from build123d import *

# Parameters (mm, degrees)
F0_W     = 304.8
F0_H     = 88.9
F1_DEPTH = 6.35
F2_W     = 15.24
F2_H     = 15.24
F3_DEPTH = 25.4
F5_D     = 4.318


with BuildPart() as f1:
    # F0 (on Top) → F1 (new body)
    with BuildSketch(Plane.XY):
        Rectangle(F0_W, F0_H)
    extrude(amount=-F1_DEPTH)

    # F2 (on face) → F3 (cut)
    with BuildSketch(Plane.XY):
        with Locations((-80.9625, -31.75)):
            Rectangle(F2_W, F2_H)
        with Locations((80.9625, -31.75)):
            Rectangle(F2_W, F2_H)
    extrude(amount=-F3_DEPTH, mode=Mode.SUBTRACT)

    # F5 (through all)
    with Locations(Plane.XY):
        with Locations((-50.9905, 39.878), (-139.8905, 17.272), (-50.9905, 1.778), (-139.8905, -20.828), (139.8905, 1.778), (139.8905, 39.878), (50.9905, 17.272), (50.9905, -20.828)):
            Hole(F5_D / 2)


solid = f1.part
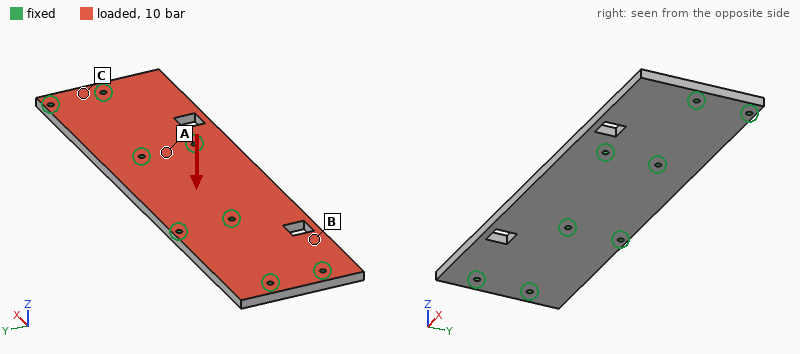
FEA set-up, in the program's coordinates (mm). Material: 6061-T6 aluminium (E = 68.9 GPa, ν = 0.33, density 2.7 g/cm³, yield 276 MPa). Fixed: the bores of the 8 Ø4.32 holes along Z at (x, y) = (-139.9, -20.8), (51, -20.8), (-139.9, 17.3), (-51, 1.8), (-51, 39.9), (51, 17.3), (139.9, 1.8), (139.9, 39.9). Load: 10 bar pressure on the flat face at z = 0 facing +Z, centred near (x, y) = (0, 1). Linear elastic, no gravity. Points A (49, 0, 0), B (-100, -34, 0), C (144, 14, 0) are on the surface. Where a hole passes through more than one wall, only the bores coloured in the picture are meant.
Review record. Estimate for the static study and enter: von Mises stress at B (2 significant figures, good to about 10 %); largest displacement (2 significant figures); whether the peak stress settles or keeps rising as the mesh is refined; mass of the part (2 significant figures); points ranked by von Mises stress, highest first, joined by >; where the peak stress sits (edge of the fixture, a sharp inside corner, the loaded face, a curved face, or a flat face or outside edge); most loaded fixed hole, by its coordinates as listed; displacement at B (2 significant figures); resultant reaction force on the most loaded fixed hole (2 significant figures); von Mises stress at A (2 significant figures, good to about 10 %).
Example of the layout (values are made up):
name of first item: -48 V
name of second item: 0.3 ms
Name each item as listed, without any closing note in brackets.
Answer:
von Mises stress at B: 41 MPa
largest displacement: 0.51 mm
whether the peak stress settles or keeps rising as the mesh is refined: keeps rising
mass of the part: 450 g
points ranked by von Mises stress, highest first, joined by >: A > B > C
where the peak stress sits: edge of the fixture
most loaded fixed hole, by its coordinates as listed: (-51, 1.8)
displacement at B: 0.27 mm
resultant reaction force on the most loaded fixed hole: 6.7 kN
von Mises stress at A: 79 MPa
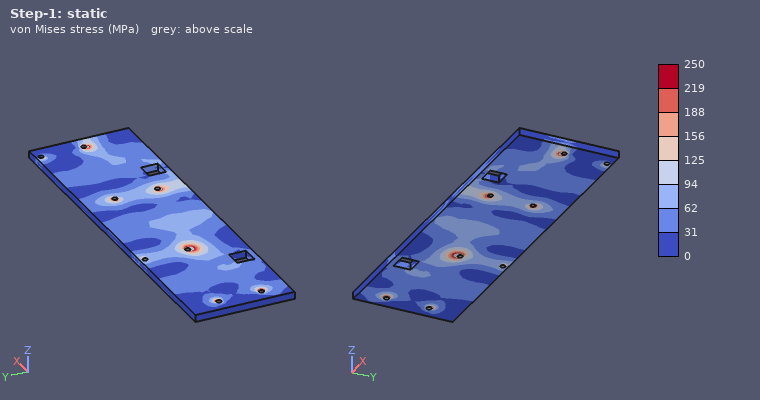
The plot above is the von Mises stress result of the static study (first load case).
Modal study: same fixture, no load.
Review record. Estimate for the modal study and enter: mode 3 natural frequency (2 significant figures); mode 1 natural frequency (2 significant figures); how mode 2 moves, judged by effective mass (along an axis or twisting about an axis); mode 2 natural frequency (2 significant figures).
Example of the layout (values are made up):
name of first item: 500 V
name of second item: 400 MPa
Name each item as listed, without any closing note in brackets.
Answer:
mode 3 natural frequency: 2700 Hz
mode 1 natural frequency: 2100 Hz
how mode 2 moves, judged by effective mass: along Z
mode 2 natural frequency: 2300 Hz
